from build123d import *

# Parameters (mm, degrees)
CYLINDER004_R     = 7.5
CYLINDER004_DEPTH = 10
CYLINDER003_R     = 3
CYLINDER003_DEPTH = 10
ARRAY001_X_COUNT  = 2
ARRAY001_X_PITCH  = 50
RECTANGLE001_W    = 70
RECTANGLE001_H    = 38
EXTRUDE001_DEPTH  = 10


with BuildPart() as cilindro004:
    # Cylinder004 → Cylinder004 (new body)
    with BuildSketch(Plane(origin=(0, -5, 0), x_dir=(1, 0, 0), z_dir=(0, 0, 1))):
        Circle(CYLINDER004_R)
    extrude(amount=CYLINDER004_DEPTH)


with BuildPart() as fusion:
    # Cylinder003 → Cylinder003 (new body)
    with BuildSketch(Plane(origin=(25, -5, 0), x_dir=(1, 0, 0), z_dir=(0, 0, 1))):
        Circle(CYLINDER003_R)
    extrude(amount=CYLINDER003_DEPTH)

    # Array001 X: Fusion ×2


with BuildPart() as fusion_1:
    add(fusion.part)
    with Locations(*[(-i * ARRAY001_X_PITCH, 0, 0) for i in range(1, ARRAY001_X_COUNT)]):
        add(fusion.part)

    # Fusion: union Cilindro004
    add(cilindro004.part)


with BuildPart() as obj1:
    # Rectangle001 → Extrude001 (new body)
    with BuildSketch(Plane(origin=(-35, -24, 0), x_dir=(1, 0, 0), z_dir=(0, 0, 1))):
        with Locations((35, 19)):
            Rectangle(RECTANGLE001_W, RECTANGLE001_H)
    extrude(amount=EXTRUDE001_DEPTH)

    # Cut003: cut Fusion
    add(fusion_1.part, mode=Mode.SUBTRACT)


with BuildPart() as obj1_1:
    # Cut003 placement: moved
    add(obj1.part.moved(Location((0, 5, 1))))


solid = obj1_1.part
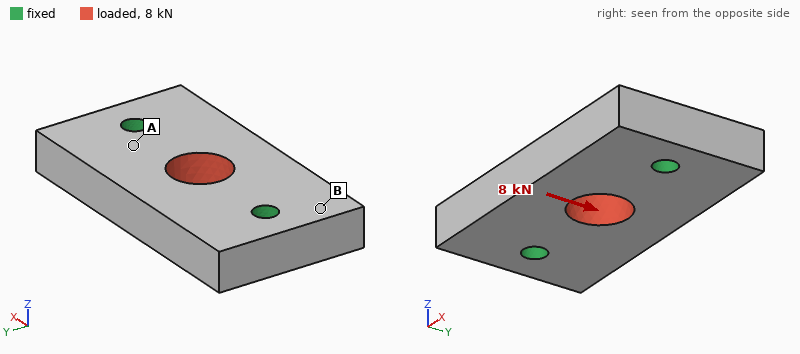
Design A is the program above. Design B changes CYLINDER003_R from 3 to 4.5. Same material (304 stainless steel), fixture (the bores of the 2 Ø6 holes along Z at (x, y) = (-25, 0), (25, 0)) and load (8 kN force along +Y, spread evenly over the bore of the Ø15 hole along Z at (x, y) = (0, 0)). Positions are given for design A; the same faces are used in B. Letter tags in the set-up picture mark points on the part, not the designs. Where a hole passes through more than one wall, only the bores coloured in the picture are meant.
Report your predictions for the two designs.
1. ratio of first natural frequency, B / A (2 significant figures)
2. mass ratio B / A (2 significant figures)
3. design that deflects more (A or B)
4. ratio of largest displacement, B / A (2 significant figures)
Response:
1.2
0.97
A
0.87
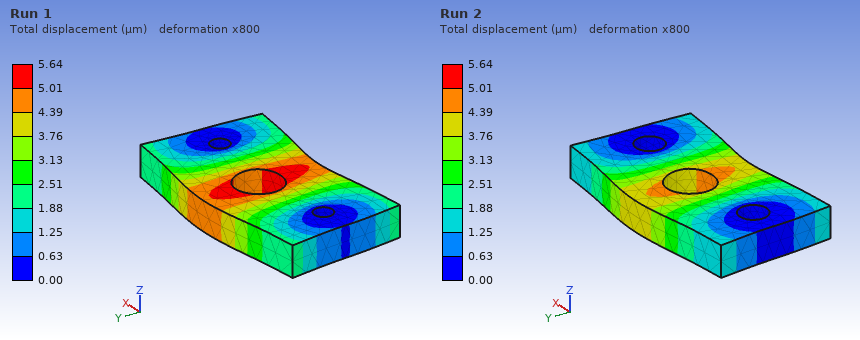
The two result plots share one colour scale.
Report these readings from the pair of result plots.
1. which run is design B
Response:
Run 2
